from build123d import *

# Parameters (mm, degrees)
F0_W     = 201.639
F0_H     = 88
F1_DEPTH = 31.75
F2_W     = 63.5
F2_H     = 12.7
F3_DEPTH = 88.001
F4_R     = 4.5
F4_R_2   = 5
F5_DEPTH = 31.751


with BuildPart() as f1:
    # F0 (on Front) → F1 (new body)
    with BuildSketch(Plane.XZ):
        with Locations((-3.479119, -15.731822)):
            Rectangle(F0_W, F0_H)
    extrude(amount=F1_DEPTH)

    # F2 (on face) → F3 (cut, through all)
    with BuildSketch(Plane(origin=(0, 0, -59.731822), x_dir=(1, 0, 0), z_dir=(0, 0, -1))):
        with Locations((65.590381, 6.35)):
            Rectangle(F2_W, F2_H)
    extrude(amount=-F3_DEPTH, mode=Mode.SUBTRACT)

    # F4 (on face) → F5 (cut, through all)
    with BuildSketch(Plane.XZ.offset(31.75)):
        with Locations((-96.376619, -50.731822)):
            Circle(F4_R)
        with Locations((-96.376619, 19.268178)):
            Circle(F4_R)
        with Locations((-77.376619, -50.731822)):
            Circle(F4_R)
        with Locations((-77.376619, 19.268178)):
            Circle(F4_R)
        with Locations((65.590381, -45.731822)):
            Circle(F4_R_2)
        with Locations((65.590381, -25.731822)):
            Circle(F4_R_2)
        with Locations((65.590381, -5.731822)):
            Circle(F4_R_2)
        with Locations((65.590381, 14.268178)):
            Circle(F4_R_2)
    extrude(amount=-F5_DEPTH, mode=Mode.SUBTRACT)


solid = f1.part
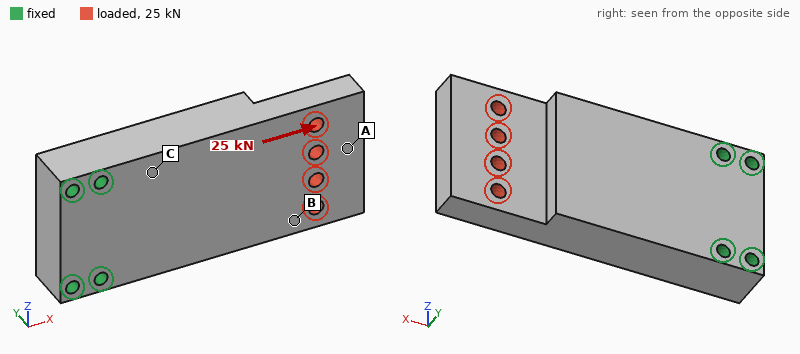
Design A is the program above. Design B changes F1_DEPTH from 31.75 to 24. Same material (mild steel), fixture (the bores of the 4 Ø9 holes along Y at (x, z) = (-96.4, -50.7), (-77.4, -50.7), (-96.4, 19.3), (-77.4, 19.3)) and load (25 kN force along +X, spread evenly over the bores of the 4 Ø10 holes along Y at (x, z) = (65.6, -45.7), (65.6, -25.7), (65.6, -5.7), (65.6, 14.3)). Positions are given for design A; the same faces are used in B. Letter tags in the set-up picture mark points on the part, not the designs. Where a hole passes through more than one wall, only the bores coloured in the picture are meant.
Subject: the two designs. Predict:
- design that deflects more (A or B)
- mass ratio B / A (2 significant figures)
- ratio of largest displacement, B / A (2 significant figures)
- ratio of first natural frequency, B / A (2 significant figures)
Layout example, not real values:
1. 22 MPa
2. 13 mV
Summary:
1. B
2. 0.72
3. 2.3
4. 0.83
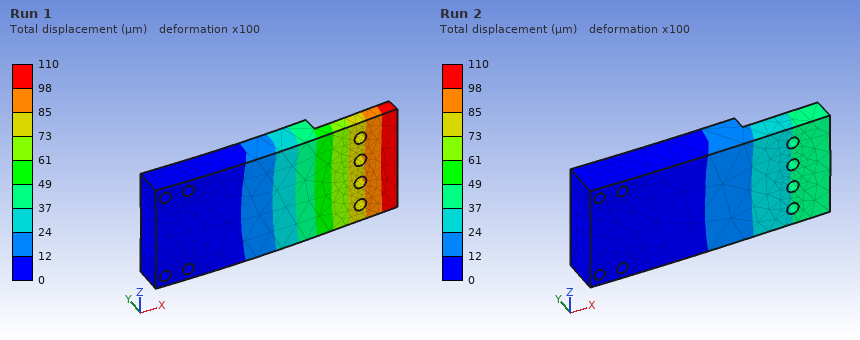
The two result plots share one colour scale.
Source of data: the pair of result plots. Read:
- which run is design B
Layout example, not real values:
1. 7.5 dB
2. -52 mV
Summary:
1. Run 1
